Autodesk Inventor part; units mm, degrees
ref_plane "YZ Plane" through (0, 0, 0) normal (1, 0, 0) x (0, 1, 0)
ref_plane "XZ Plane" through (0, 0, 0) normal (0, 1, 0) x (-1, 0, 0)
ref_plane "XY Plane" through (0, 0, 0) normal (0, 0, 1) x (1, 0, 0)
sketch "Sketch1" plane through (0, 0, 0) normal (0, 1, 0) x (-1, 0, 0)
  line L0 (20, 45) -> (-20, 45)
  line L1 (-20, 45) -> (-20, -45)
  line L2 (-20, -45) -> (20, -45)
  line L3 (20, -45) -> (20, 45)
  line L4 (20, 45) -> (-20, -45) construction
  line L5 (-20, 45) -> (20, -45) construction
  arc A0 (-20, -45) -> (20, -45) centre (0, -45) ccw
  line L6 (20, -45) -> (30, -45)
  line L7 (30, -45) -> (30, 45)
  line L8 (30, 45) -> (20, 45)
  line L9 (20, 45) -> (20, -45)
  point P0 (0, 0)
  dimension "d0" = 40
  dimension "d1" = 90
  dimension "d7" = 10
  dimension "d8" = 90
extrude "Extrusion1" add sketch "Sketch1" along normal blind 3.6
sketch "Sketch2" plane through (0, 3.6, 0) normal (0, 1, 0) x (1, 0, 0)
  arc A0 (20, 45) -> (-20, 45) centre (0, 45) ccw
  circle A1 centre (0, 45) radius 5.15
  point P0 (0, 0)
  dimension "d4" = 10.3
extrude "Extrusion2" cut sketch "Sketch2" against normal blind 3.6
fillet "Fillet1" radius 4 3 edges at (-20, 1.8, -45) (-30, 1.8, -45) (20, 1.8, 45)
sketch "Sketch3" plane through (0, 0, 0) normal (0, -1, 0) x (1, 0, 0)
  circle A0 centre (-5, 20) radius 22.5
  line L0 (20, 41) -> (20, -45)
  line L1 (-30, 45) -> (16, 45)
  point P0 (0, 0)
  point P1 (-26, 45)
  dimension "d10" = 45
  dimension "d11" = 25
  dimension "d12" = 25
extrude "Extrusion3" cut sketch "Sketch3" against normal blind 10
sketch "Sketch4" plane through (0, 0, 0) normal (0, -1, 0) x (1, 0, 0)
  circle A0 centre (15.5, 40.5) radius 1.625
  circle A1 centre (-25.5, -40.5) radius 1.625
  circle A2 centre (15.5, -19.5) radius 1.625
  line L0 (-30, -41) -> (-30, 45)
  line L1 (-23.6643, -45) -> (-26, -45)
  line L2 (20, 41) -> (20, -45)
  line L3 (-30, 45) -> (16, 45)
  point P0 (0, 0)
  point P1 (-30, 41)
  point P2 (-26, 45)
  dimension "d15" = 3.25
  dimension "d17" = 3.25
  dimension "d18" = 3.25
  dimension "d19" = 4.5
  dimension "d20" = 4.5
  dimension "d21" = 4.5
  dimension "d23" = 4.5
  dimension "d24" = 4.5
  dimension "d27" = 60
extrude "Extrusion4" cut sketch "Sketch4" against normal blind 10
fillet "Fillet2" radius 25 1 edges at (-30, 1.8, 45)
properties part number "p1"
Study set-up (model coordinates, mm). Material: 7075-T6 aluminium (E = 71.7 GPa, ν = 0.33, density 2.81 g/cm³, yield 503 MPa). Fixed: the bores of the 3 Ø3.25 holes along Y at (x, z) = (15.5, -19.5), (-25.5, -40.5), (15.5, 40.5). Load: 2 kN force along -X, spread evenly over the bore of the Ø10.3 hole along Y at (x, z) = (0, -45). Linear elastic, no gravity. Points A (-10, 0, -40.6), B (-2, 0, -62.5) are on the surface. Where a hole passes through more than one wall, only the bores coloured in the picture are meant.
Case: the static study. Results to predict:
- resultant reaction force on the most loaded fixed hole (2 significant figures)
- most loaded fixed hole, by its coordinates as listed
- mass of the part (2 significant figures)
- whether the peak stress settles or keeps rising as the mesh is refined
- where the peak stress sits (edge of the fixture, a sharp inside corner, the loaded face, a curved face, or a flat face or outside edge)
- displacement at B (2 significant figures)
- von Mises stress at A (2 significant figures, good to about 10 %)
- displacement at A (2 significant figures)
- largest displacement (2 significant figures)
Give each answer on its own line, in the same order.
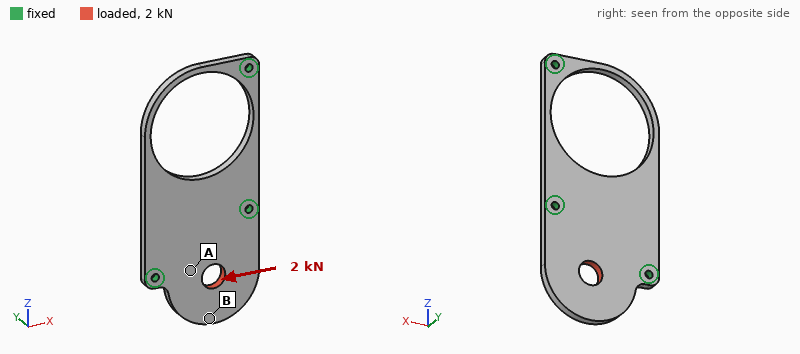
1.5 kN
(-25.5, -40.5)
33 g
keeps rising
edge of the fixture
14 µm
23 MPa
6.0 µm
15 µm
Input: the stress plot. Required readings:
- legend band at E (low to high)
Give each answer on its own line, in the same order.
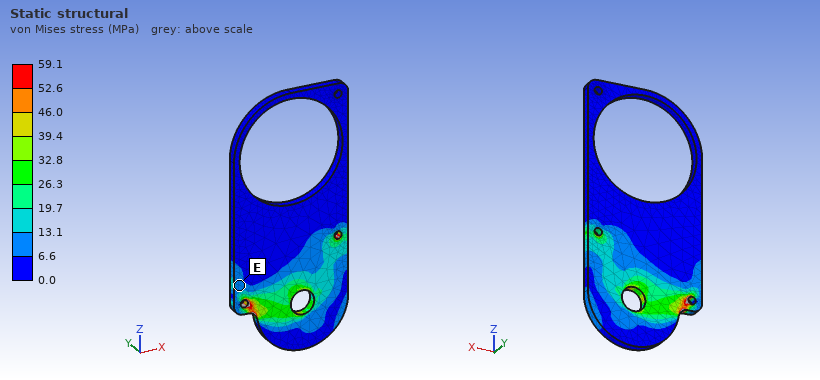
6.6 to 13.1 MPa
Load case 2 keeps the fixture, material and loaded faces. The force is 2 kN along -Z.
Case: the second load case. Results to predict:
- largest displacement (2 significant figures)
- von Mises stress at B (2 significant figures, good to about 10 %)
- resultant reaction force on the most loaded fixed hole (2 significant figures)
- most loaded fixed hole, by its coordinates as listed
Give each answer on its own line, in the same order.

11 µm
9.0 MPa
1.2 kN
(15.5, -19.5)
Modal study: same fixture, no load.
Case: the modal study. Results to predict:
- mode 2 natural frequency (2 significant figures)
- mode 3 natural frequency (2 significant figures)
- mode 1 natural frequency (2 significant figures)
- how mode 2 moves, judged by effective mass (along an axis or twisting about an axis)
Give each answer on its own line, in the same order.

2400 Hz
3800 Hz
1800 Hz
along Y
